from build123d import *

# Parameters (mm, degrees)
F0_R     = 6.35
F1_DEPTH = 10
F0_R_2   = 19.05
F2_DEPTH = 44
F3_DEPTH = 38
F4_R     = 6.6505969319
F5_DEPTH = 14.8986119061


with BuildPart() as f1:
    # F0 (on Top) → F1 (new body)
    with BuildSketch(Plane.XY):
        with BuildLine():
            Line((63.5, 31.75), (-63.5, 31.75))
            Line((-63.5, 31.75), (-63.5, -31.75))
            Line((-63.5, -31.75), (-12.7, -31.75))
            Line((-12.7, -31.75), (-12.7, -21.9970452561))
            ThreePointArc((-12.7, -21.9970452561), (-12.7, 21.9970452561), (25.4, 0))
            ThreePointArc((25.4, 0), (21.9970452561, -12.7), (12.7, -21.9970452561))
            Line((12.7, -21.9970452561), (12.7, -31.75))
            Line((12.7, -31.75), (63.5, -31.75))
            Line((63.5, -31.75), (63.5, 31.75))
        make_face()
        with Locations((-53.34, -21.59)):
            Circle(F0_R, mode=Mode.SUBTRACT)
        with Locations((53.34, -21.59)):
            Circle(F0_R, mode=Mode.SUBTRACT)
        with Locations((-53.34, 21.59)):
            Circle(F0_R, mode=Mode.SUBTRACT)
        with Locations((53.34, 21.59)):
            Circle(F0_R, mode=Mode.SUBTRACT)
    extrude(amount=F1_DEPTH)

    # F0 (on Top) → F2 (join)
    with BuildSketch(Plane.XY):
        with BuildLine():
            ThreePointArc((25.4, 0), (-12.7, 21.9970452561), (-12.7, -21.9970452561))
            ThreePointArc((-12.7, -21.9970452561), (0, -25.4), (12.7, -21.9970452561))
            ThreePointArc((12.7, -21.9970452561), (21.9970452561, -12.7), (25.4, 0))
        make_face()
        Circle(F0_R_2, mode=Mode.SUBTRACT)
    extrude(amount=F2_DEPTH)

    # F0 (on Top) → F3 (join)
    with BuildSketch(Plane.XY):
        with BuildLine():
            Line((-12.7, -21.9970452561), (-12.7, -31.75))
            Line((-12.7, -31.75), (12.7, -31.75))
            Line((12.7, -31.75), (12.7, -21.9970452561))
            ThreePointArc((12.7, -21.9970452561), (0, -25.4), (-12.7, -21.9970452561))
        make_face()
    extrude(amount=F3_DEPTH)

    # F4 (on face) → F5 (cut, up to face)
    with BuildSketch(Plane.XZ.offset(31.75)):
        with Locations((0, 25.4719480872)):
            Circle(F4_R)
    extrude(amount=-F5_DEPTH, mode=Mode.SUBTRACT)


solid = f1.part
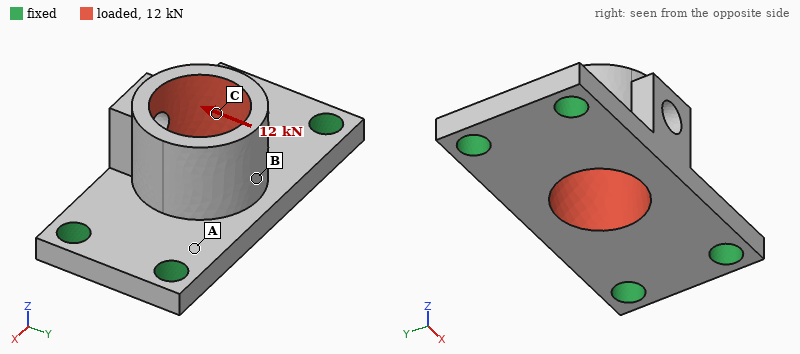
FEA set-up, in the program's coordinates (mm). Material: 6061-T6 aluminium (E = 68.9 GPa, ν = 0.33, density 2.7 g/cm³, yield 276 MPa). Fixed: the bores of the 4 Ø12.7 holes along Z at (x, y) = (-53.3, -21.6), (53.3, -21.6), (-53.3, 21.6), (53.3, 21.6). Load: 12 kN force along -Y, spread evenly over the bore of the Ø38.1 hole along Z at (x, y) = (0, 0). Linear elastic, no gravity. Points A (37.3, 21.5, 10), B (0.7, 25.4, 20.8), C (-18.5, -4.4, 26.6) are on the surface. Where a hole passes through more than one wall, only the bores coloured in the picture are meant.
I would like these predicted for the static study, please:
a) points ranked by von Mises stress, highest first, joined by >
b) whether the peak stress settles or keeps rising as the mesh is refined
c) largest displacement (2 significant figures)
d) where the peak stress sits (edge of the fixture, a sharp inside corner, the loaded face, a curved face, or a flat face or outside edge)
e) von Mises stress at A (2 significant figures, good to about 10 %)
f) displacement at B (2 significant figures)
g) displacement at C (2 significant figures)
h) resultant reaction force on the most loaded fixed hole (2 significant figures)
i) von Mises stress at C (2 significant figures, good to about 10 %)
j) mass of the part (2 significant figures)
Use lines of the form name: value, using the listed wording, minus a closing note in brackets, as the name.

points ranked by von Mises stress, highest first, joined by >: A > C > B
whether the peak stress settles or keeps rising as the mesh is refined: keeps rising
largest displacement: 0.18 mm
where the peak stress sits: edge of the fixture
von Mises stress at A: 49 MPa
displacement at B: 0.11 mm
displacement at C: 0.087 mm
resultant reaction force on the most loaded fixed hole: 4.8 kN
von Mises stress at C: 27 MPa
mass of the part: 260 g
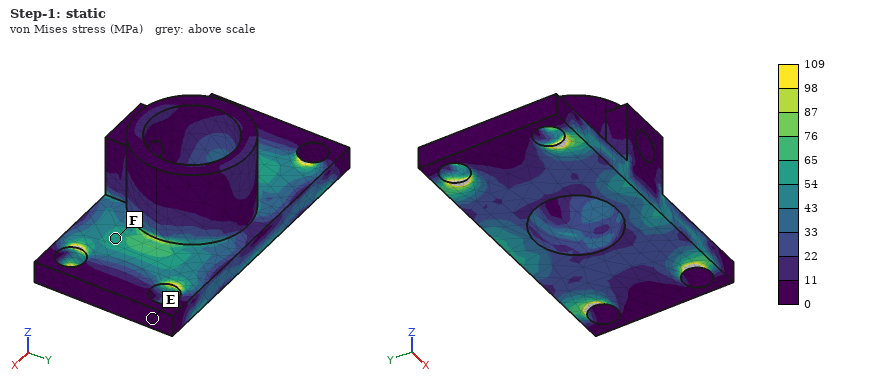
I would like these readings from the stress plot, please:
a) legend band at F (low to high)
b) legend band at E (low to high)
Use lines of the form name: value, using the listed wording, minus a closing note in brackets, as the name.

legend band at F: 54 to 65 MPa
legend band at E: 0 to 11 MPa
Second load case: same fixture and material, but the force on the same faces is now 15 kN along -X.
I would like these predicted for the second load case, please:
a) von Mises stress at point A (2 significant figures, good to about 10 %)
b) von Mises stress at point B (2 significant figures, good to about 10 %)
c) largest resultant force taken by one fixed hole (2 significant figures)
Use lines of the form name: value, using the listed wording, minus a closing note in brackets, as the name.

von Mises stress at point A: 13 MPa
von Mises stress at point B: 18 MPa
largest resultant force taken by one fixed hole: 4.2 kN
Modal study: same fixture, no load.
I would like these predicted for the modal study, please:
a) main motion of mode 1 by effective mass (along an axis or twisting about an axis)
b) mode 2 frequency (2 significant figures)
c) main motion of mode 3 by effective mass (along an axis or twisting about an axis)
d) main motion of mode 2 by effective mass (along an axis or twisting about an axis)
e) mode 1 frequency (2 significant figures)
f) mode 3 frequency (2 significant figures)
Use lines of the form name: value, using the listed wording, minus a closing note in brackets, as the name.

main motion of mode 1 by effective mass: along Y
mode 2 frequency: 4500 Hz
main motion of mode 3 by effective mass: along X
main motion of mode 2 by effective mass: along Z
mode 1 frequency: 3800 Hz
mode 3 frequency: 6500 Hz
